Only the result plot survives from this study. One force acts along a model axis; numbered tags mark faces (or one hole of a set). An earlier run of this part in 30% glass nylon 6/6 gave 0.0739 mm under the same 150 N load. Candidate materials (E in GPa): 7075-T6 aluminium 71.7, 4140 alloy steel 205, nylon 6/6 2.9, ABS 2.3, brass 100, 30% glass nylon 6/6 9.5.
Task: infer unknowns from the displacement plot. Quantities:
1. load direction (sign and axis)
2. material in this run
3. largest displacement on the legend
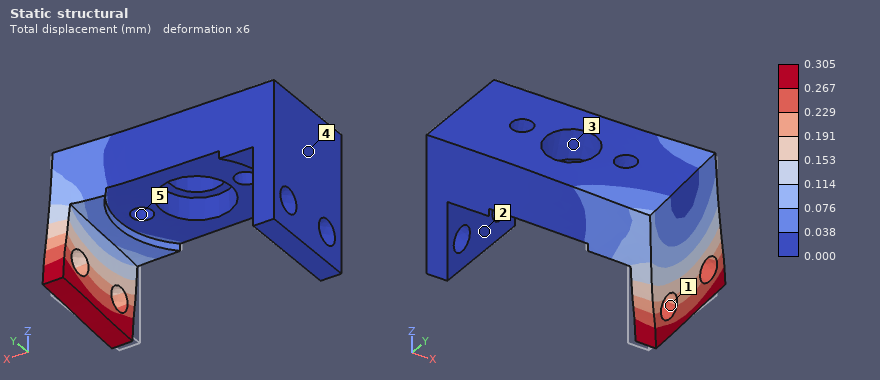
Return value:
+Y
ABS
0.305 mm
